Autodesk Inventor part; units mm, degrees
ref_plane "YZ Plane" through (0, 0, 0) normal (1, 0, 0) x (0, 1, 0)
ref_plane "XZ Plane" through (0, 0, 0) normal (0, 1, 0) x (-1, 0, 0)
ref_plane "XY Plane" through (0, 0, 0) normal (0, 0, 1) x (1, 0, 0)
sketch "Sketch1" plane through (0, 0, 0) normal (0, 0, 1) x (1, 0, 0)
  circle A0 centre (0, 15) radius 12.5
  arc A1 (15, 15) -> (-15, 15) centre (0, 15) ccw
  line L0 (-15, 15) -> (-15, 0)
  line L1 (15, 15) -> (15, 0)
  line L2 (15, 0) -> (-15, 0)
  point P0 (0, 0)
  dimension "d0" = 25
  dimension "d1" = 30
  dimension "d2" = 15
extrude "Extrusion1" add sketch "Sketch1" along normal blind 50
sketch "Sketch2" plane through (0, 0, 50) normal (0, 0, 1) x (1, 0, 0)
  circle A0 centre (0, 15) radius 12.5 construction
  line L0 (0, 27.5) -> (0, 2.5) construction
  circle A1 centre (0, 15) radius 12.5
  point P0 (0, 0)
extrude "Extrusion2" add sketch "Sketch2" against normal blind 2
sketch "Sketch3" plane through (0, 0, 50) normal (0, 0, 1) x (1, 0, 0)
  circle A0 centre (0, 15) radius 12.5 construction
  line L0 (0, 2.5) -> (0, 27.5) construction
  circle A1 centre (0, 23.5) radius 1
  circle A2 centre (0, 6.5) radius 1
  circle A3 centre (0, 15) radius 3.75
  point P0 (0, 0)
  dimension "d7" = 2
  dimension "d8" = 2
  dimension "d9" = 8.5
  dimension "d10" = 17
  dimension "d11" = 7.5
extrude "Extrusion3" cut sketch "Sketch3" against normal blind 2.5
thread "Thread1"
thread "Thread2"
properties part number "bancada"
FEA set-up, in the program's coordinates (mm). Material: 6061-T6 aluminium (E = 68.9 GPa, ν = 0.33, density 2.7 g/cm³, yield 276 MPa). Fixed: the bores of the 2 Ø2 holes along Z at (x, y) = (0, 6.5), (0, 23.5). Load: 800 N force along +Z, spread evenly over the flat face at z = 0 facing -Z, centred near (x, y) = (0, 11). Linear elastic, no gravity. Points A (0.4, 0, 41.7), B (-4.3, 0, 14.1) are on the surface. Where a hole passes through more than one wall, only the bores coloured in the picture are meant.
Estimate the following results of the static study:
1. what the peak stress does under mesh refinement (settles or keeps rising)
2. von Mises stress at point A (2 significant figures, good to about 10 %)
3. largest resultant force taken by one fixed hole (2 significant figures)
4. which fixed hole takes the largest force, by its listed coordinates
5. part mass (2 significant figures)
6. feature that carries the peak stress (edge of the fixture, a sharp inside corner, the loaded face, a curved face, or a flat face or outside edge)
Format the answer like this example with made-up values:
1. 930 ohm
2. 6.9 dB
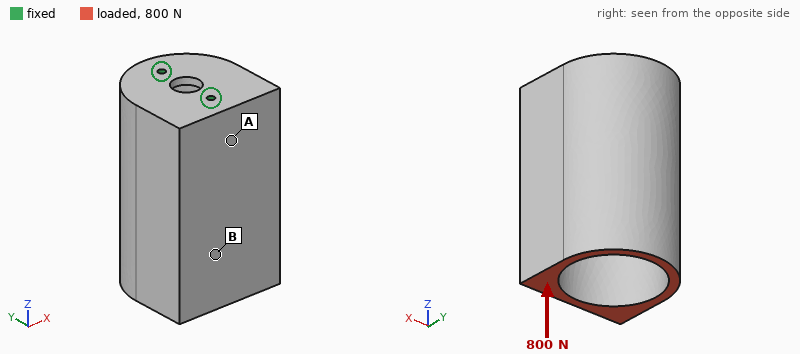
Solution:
1. keeps rising
2. 13 MPa
3. 540 N
4. (0, 6.5)
5. 45 g
6. edge of the fixture
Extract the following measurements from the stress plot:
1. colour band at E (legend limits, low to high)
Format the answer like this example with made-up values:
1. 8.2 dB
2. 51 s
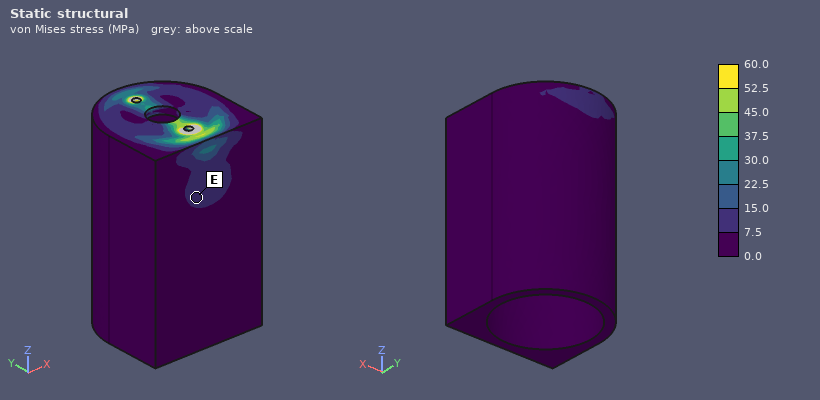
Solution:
1. 7.5 to 15.0 MPa
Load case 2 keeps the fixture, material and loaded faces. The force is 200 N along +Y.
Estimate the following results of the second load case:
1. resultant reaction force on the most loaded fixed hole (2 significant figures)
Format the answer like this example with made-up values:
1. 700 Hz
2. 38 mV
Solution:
1. 480 N
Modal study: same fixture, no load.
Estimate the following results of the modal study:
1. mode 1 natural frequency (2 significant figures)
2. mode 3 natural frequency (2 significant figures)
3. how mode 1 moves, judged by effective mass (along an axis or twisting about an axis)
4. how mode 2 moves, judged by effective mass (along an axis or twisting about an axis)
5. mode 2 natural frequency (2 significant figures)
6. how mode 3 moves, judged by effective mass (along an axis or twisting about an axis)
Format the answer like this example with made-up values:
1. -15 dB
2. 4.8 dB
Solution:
1. 660 Hz
2. 6100 Hz
3. along X
4. along Y
5. 2000 Hz
6. along Z
